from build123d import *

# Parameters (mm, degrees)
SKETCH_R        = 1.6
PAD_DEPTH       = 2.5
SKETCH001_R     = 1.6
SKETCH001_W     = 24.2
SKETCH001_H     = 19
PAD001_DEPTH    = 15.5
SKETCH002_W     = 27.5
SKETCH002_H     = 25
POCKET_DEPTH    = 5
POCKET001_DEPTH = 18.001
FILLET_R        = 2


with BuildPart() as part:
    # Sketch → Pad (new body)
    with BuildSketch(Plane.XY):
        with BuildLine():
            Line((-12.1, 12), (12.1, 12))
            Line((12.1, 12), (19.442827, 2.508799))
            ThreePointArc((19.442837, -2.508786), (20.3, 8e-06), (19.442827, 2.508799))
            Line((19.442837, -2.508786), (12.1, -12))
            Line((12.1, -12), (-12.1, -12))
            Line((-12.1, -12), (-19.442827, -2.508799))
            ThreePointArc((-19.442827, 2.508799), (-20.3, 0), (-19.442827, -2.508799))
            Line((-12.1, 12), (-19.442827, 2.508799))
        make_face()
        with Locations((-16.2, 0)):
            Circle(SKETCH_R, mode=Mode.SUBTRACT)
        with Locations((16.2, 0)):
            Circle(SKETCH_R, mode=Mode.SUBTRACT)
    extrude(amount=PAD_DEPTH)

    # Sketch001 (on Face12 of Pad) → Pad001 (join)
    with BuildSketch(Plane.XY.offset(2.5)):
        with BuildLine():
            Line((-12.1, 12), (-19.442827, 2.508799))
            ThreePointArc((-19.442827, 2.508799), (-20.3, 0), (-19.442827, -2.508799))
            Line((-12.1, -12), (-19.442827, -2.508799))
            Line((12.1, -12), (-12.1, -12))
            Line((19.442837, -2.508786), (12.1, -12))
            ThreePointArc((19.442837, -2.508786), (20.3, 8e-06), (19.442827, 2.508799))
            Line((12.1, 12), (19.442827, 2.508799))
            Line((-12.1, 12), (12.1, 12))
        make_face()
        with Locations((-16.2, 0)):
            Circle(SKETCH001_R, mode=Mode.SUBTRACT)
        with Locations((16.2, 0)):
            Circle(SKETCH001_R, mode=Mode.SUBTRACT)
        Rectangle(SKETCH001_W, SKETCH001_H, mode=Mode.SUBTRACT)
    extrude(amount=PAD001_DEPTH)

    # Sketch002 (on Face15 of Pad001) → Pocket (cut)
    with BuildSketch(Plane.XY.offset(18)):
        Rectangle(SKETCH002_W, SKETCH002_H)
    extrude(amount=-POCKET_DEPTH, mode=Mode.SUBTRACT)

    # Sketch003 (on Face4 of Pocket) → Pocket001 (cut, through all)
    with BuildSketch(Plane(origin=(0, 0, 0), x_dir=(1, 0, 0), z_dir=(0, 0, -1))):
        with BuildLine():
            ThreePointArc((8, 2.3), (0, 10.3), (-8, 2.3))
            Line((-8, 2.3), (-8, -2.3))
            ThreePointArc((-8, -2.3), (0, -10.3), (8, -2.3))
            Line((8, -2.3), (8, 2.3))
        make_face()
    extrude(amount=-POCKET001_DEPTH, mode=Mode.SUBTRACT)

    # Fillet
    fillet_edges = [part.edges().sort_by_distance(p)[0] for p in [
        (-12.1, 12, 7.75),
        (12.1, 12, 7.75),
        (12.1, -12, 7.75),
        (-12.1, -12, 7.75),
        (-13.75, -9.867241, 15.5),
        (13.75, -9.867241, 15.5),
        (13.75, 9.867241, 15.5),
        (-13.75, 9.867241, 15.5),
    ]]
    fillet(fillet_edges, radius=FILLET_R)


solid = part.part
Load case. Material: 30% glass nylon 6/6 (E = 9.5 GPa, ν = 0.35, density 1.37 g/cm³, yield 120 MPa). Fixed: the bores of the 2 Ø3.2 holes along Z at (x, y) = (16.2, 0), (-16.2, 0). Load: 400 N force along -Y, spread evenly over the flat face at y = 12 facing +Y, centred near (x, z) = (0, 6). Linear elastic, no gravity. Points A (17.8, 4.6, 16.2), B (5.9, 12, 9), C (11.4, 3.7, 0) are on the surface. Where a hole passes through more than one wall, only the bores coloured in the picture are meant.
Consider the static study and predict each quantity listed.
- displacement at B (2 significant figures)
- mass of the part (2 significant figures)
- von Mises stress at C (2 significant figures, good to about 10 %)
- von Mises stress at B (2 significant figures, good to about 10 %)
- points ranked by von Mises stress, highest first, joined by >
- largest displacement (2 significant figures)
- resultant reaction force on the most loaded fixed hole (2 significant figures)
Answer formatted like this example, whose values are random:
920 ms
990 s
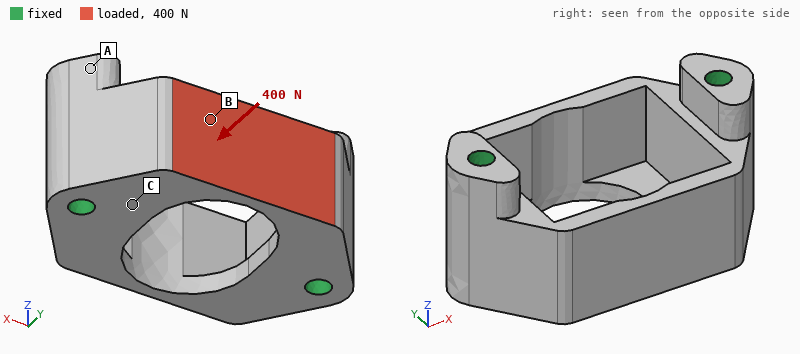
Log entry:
0.100 mm
7.0 g
13 MPa
23 MPa
B > C > A
0.21 mm
280 N
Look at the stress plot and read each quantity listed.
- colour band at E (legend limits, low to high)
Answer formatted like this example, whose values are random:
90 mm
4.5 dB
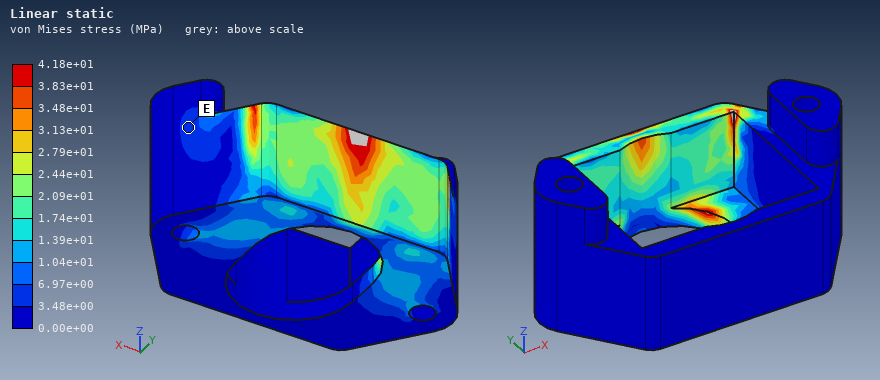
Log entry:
3.48e+00 to 6.97e+00 MPa
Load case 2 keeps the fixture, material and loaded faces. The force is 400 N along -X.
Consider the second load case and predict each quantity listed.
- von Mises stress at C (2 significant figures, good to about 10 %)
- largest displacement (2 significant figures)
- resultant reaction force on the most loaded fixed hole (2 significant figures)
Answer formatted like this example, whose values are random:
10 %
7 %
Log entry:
5.2 MPa
39 µm
210 N
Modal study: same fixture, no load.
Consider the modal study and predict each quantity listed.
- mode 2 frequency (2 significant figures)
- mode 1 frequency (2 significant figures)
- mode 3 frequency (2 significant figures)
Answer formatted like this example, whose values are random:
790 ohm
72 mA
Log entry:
10 kHz
10 kHz
13 kHz
